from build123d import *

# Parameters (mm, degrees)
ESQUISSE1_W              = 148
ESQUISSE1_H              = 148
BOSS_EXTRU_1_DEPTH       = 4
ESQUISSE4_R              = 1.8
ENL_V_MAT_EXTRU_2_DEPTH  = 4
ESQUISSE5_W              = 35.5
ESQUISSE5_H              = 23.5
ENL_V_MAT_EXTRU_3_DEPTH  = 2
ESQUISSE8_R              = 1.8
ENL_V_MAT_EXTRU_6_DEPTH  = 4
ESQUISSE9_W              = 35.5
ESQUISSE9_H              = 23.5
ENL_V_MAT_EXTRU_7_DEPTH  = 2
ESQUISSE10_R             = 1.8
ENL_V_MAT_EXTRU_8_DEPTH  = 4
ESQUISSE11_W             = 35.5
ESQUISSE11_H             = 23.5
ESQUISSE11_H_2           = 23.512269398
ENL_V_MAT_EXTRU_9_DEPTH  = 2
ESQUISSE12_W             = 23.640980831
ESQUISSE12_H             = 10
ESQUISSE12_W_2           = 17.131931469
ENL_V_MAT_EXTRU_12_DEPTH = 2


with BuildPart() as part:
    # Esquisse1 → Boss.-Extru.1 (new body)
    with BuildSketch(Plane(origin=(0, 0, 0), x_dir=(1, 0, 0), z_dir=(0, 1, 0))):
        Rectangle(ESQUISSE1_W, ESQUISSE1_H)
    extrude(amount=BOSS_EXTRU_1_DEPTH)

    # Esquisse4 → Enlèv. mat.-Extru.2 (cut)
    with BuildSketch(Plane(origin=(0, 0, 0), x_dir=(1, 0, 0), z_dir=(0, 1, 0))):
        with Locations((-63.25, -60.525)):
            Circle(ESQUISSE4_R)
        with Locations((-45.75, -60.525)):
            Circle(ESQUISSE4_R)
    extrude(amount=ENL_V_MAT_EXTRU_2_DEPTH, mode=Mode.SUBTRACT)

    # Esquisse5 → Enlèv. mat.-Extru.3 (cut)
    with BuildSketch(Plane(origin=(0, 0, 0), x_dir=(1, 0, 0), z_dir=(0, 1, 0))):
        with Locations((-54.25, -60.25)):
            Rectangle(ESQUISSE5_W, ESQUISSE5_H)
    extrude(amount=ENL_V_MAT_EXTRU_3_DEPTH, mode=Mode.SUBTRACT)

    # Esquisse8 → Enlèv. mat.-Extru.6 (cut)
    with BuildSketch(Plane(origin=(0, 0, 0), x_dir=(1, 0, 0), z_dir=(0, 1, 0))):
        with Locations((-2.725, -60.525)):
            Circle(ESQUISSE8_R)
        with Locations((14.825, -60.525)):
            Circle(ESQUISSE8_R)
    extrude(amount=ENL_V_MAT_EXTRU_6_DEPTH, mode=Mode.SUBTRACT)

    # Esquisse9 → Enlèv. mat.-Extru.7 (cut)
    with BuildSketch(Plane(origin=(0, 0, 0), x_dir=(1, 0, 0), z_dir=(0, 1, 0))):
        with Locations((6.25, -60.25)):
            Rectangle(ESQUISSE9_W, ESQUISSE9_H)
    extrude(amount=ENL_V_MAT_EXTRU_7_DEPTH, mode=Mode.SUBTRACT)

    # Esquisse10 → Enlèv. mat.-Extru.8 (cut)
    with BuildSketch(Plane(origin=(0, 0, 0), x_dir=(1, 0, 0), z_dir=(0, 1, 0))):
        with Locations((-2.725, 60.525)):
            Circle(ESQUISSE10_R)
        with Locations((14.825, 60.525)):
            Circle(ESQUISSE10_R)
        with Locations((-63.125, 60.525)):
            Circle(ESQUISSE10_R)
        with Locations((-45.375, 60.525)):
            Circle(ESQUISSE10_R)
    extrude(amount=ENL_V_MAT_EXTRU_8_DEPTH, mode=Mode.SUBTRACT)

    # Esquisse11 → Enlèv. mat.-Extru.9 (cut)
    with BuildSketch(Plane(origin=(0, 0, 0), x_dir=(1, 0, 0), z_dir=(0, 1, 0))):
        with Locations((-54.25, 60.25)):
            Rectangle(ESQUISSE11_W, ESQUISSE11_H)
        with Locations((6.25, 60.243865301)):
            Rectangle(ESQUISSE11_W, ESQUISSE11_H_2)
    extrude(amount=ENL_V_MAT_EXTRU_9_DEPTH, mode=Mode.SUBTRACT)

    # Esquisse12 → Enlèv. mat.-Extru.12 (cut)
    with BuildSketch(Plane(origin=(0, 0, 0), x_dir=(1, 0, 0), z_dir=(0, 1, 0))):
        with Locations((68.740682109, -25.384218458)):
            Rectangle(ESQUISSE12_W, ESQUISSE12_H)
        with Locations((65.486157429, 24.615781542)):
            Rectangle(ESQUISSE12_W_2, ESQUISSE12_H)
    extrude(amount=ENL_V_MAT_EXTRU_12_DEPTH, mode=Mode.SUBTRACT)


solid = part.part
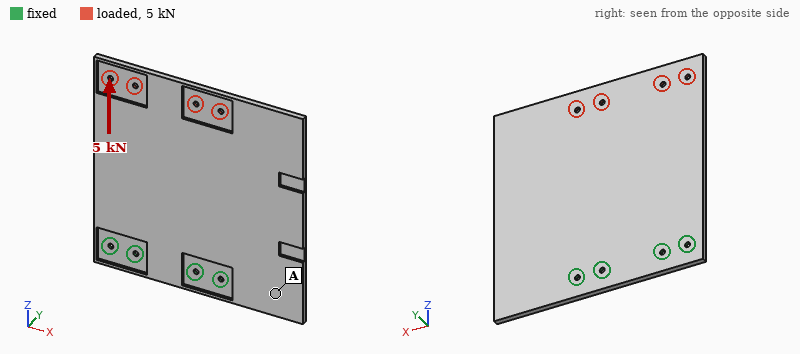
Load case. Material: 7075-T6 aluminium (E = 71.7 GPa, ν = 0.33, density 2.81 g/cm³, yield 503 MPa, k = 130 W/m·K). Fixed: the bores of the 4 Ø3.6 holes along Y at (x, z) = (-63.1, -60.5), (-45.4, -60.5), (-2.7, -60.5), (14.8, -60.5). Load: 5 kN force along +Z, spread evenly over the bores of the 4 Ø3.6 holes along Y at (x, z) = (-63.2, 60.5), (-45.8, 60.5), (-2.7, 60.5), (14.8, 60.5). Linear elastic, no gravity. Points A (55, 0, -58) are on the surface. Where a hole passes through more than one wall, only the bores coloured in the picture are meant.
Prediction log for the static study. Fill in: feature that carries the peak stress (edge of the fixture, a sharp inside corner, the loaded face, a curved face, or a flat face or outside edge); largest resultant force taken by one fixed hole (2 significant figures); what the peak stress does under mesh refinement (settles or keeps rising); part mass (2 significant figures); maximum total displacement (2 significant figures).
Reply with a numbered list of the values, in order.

1. edge of the fixture
2. 1.3 kN
3. keeps rising
4. 230 g
5. 0.73 mm
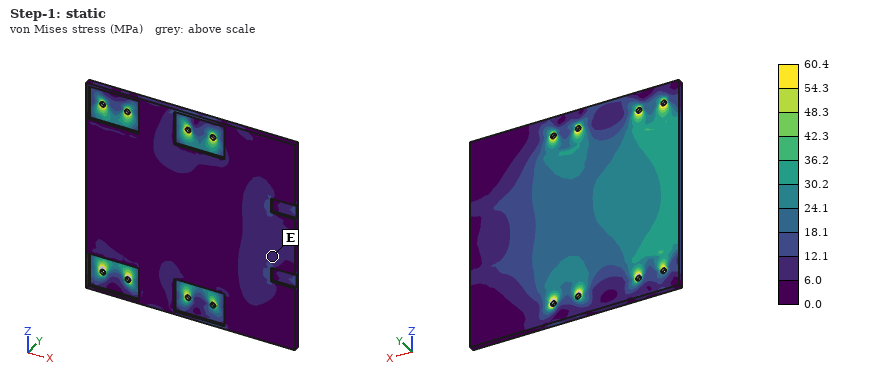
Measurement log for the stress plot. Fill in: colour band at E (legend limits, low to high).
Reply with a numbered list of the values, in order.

1. 6.0 to 12.1 MPa
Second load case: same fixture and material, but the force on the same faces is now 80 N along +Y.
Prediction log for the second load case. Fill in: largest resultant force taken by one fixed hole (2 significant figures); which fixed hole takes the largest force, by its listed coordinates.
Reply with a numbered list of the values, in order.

1. 110 N
2. (-45.4, -60.5)
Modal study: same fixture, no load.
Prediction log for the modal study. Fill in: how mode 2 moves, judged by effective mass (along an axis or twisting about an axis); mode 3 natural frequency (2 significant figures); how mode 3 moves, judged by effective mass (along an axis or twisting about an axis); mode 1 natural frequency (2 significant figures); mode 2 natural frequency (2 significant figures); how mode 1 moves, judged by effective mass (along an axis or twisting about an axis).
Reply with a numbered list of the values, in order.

1. twisting about Z
2. 690 Hz
3. along Y
4. 120 Hz
5. 300 Hz
6. along Y
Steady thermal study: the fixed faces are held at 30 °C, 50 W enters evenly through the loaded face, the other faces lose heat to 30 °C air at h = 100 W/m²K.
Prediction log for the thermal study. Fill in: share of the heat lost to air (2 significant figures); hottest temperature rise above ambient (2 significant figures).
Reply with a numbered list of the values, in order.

1. 92 %
2. 51 K
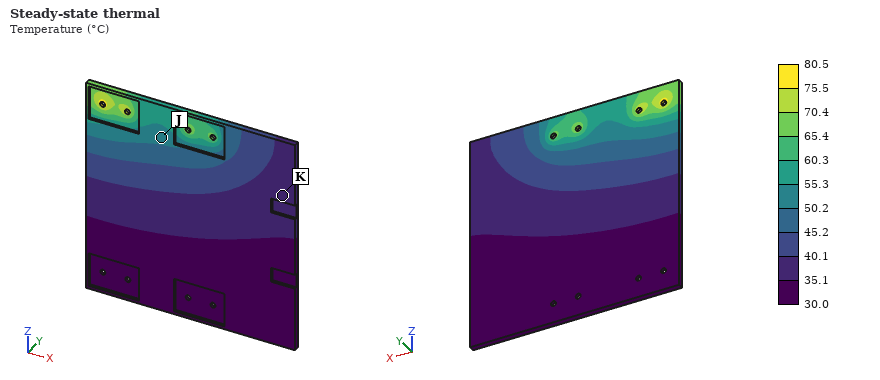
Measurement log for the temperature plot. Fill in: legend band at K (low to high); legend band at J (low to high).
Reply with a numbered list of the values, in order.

1. 35.1 to 40.1 °C
2. 50.2 to 55.3 °C
